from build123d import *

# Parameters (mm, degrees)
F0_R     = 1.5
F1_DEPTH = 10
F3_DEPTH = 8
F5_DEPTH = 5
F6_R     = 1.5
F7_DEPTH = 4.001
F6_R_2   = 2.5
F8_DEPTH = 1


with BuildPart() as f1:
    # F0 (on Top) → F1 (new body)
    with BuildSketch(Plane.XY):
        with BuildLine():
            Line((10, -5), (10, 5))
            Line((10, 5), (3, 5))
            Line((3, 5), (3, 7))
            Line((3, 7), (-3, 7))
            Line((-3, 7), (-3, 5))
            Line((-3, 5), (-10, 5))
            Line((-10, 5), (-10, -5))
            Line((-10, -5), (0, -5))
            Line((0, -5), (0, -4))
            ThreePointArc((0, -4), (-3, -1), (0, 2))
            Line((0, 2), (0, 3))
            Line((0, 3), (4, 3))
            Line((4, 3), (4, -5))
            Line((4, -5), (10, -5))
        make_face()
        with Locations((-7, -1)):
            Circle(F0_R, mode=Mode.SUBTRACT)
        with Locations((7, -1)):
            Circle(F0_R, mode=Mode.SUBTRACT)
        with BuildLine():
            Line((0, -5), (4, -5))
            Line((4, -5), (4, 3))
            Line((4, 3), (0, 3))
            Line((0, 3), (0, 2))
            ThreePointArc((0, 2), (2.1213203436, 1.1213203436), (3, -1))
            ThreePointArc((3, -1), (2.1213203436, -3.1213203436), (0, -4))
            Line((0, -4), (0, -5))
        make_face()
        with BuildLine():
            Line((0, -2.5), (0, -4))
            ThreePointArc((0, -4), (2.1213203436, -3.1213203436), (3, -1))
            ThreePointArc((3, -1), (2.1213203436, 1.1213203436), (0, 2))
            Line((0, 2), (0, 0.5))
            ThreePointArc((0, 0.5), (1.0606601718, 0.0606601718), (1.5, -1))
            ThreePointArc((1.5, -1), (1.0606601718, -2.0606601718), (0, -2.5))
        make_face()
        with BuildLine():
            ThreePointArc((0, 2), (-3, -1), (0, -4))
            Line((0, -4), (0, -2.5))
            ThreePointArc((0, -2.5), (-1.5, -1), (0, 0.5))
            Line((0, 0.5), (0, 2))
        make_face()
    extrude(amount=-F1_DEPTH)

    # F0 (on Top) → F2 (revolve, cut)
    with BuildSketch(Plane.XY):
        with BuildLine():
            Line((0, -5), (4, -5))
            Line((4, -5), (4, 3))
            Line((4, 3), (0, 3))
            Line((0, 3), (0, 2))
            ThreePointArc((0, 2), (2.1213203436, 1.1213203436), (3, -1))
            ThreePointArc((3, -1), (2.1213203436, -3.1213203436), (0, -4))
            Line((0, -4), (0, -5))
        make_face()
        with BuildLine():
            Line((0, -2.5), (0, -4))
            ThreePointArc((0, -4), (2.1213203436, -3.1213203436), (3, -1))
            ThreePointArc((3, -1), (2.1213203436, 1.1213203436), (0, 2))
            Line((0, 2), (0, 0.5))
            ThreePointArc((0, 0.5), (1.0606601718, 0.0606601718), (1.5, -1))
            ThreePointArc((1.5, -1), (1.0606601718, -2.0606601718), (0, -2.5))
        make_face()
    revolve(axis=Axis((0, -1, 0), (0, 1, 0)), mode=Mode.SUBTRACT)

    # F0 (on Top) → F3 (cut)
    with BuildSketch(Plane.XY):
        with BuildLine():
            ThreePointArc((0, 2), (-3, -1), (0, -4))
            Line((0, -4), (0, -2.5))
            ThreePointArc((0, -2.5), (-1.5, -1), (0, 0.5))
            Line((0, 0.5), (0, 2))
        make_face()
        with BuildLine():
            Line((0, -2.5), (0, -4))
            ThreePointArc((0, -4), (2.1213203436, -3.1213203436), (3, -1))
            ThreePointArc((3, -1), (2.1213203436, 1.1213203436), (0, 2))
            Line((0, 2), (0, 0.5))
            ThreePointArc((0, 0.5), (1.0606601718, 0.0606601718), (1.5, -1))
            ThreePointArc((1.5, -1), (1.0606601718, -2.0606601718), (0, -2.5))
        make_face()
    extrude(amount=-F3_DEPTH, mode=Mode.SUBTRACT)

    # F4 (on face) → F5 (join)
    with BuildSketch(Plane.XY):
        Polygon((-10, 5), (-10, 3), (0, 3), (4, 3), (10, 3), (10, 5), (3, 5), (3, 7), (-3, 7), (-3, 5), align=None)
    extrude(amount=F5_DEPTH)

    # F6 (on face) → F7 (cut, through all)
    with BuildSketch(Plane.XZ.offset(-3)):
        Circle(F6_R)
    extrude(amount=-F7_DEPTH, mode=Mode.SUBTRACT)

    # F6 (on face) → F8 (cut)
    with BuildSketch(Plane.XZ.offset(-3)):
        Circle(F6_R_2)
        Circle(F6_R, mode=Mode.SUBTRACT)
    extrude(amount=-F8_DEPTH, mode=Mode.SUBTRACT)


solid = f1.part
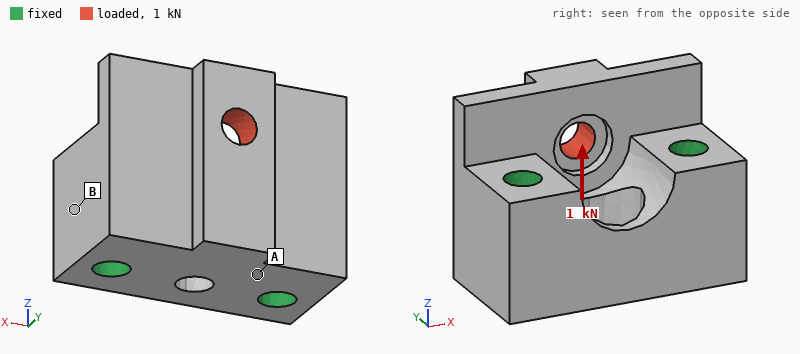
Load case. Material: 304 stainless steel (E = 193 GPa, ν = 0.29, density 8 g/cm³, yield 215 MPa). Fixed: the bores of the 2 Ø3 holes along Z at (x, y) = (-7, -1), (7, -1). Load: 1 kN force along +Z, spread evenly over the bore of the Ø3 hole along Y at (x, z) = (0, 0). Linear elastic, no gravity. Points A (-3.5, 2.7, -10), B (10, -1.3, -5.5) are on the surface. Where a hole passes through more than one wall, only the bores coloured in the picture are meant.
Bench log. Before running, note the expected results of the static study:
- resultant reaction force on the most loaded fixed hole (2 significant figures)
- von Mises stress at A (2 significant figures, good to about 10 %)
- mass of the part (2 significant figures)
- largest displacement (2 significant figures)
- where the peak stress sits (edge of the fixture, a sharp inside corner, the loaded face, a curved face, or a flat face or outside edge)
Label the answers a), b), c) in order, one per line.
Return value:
a) 500 N
b) 21 MPa
c) 15 g
d) 6.3 µm
e) the loaded face
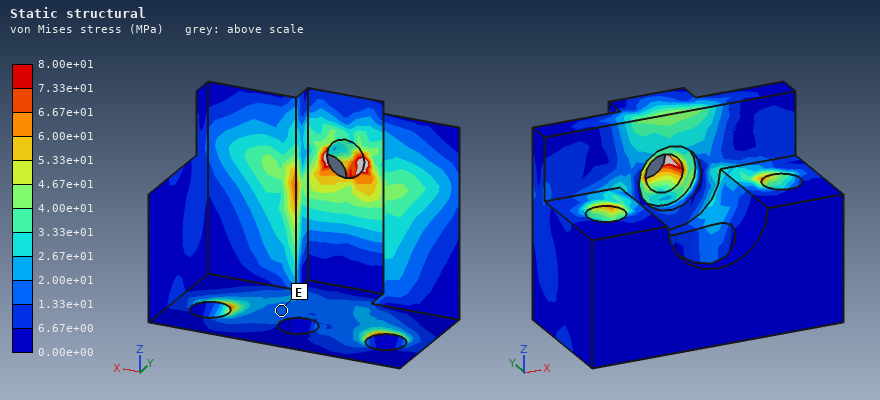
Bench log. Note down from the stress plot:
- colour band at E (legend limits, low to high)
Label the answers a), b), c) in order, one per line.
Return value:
a) 1.33e+01 to 2.00e+01 MPa
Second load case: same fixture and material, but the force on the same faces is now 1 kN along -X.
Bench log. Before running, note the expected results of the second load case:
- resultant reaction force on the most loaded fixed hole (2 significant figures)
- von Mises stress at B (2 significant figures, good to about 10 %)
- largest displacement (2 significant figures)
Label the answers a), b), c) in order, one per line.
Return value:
a) 640 N
b) 7.7 MPa
c) 3.1 µm
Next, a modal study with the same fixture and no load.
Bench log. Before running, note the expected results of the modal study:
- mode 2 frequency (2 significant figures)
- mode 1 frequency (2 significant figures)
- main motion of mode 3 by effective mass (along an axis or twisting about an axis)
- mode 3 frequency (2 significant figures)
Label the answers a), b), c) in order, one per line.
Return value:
a) 48 kHz
b) 34 kHz
c) along X
d) 60 kHz
